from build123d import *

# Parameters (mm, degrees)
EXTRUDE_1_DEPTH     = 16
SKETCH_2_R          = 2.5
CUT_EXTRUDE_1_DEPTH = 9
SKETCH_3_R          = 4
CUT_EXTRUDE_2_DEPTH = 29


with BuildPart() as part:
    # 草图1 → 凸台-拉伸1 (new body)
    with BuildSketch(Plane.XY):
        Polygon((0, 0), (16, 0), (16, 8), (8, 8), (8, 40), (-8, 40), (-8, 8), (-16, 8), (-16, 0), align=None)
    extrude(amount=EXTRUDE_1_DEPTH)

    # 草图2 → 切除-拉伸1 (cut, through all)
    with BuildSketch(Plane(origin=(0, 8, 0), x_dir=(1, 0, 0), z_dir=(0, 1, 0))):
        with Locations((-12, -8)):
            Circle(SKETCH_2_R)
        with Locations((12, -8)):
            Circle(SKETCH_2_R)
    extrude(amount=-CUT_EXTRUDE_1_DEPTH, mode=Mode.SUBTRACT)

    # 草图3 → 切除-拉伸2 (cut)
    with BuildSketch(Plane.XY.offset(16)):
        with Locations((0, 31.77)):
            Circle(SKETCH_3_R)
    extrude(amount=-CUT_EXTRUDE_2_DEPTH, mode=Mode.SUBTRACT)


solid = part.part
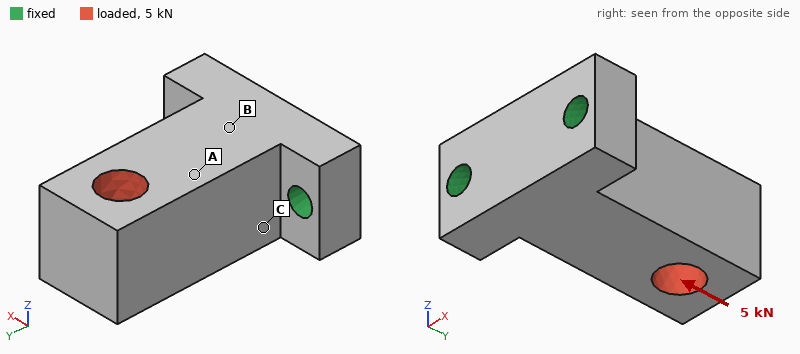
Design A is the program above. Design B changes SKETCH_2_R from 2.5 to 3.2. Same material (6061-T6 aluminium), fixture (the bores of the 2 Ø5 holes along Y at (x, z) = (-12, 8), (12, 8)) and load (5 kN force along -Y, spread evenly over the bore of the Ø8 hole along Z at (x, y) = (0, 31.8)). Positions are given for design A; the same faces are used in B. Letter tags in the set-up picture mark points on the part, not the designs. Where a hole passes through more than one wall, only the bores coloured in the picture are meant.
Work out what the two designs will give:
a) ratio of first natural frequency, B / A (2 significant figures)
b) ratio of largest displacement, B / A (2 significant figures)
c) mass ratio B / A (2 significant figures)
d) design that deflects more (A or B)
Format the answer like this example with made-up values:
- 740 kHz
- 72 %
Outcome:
- 1.1
- 0.92
- 0.98
- A
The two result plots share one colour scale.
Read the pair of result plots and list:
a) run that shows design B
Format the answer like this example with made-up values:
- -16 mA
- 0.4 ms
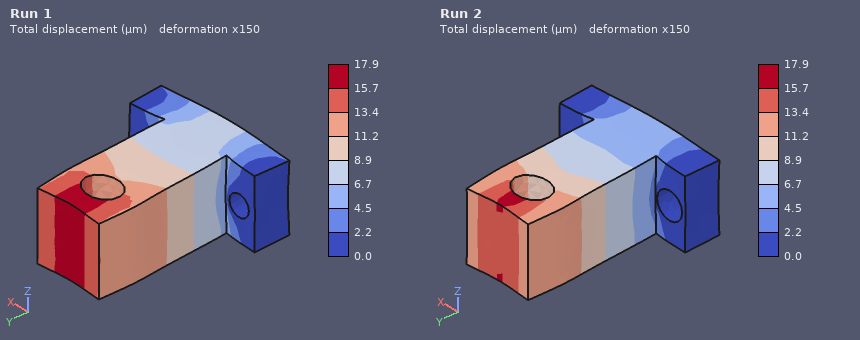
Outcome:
- Run 2
